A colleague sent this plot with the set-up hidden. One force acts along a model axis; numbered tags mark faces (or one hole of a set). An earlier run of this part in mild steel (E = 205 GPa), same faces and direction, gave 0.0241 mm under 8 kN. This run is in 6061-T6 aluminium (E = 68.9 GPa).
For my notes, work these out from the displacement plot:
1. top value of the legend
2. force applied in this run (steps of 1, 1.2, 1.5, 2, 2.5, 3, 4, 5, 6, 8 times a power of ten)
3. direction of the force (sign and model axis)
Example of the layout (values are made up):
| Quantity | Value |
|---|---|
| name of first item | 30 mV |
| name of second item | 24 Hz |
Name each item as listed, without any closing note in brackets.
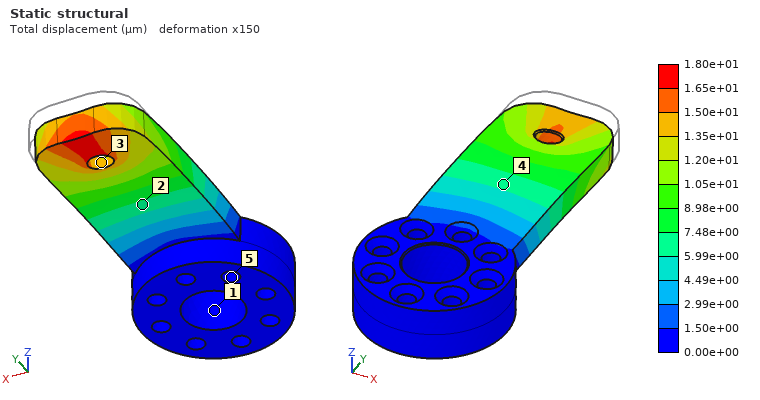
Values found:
| Quantity | Value |
|---|---|
| top value of the legend | 1.80e+01 µm |
| force applied in this run | 2 kN |
| direction of the force | -Y |
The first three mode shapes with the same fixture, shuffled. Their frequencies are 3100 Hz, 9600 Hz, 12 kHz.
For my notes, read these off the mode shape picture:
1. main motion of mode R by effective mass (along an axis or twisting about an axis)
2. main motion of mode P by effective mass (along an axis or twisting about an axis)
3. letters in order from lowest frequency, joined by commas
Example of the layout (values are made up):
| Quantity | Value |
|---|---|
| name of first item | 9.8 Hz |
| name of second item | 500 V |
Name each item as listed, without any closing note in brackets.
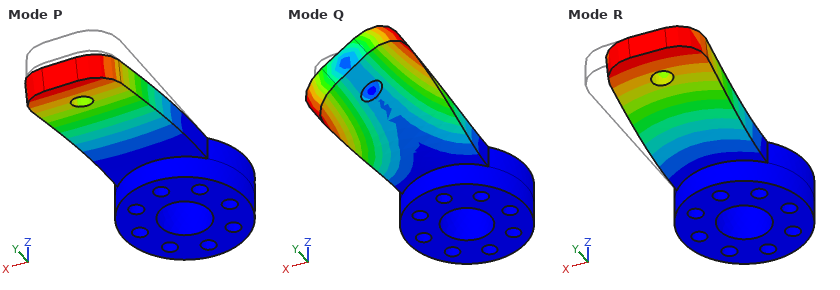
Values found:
| Quantity | Value |
|---|---|
| main motion of mode R by effective mass | along X |
| main motion of mode P by effective mass | along Z |
| letters in order from lowest frequency, joined by commas | P, R, Q |
